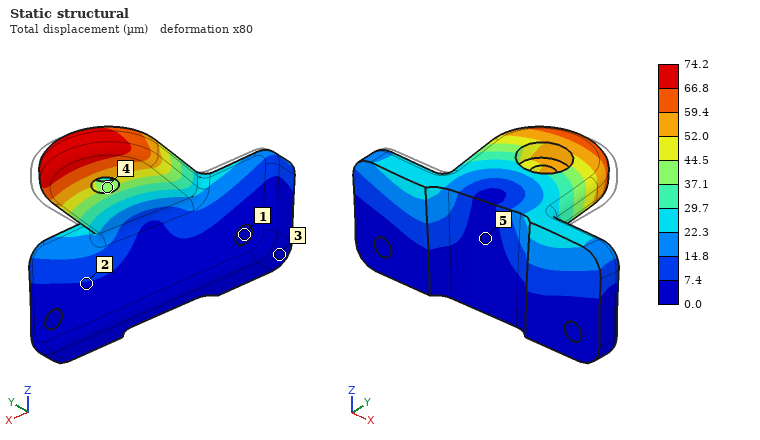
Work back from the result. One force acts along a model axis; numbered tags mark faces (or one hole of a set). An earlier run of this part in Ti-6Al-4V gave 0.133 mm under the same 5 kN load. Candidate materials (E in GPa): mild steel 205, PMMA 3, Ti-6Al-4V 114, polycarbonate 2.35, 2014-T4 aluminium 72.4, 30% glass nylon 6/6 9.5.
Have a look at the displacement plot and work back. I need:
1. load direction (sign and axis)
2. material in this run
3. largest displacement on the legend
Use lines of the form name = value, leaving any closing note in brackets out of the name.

load direction = -X
material in this run = mild steel
largest displacement on the legend = 74.2 µm
